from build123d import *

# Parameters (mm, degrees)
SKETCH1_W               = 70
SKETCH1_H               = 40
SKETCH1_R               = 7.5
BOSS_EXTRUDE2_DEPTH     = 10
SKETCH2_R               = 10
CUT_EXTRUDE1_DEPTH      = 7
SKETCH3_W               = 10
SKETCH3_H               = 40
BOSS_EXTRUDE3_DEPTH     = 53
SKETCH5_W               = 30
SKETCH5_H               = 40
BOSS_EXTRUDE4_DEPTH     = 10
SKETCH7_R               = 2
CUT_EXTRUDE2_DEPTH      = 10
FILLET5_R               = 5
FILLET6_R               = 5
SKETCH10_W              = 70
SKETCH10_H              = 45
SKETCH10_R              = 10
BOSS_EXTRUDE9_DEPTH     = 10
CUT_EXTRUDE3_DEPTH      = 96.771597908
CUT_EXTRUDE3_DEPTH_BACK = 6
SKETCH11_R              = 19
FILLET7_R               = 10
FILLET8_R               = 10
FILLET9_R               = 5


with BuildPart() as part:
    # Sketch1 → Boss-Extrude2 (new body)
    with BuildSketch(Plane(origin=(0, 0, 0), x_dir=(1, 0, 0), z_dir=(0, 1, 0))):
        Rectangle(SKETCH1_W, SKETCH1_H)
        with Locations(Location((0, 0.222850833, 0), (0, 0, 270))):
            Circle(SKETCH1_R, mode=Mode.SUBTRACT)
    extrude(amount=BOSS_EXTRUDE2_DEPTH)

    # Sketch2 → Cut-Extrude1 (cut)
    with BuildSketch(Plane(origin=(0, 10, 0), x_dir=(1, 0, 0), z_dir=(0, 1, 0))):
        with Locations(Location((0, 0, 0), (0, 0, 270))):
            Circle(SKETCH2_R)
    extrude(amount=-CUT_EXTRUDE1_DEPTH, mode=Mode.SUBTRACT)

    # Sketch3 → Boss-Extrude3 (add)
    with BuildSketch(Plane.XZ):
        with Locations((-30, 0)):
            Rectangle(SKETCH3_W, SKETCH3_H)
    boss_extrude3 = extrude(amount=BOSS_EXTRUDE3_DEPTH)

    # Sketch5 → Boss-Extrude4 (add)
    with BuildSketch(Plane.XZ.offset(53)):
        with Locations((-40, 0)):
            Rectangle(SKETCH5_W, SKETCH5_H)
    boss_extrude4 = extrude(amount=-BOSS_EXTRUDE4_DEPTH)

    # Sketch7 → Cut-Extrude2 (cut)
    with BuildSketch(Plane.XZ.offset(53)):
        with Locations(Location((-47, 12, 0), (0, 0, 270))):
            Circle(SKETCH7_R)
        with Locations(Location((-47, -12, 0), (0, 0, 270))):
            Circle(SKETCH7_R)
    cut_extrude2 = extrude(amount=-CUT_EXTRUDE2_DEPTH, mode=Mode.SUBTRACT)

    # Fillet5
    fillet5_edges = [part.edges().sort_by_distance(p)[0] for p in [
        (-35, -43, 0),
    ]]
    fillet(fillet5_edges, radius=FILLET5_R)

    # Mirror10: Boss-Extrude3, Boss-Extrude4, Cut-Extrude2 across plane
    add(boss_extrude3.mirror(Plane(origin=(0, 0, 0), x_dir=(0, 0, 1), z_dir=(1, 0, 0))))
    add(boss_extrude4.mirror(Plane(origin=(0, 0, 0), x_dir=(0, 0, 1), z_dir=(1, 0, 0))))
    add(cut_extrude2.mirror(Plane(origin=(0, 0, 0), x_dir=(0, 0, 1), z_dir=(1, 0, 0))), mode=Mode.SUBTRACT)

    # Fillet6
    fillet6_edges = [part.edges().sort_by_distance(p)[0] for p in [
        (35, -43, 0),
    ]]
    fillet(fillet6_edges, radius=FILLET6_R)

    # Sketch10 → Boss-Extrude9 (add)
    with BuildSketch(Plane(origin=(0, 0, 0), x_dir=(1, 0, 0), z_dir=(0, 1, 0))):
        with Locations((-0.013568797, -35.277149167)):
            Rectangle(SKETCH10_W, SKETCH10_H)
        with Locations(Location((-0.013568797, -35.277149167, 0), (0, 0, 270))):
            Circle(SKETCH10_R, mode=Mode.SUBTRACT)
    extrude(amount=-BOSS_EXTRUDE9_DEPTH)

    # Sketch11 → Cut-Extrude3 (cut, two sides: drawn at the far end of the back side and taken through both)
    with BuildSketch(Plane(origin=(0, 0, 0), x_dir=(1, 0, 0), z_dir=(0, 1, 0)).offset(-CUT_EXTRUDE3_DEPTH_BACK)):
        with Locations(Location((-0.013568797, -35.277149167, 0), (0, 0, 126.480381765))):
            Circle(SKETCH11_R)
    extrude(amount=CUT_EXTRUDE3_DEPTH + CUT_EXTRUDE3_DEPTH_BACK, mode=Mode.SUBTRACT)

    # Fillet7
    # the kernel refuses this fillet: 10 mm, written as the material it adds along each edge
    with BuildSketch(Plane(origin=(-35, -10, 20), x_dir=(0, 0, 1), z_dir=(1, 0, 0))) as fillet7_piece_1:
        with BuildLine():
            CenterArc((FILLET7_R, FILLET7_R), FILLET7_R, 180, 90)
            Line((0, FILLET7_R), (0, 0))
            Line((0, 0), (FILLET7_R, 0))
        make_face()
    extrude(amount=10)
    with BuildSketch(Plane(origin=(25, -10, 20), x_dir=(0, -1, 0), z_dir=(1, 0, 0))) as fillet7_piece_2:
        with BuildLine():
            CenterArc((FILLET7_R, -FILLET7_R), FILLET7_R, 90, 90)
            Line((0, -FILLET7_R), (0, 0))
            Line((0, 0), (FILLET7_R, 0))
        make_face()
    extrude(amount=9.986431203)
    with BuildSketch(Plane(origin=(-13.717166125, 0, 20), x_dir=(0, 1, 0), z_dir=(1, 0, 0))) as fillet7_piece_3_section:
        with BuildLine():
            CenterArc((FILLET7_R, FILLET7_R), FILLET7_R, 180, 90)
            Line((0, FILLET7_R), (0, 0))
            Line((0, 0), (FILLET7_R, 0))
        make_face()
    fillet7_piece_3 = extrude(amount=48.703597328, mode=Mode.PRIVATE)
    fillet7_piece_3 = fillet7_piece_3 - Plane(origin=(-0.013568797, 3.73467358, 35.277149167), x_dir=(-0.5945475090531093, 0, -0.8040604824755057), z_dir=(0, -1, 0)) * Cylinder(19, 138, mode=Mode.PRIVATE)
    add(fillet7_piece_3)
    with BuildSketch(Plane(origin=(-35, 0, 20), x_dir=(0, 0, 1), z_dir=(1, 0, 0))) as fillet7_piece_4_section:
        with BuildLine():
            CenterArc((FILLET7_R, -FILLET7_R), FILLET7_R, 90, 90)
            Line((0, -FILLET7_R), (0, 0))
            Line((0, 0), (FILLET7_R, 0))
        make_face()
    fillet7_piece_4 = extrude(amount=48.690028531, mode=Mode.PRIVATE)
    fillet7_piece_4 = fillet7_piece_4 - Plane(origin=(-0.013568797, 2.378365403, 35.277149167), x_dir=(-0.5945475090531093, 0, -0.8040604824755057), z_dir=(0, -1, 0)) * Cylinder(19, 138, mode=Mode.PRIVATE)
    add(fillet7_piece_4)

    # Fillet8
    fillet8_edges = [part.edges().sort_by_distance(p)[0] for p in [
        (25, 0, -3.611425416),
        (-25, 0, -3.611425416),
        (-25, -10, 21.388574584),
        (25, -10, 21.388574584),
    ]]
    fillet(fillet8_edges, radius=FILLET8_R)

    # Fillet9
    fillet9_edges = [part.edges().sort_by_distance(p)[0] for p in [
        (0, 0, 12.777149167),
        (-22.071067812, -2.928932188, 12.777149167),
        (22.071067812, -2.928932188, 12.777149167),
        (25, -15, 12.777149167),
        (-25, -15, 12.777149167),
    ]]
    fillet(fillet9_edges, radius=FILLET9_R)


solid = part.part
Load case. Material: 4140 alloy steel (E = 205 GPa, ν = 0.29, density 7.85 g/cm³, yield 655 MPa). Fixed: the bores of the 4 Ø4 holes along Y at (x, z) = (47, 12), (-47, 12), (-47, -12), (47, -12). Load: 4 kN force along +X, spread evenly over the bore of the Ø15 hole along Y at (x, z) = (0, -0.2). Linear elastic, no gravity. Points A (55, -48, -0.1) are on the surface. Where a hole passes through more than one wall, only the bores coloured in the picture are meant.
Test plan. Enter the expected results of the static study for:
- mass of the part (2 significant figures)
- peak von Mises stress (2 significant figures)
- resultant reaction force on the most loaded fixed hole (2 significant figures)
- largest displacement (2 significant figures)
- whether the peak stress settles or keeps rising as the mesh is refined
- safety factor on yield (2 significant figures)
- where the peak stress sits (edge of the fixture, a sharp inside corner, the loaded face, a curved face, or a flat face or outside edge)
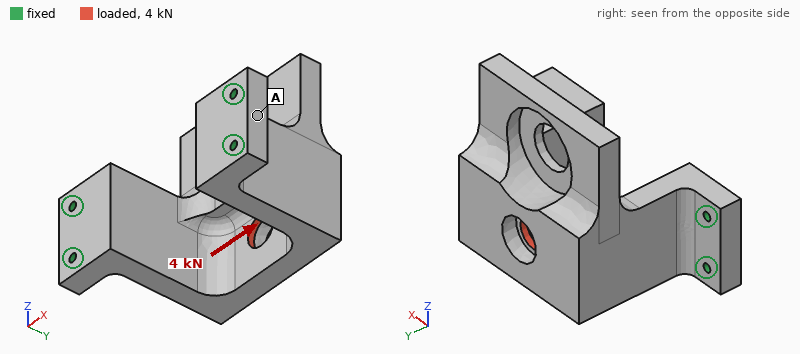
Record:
850 g
91 MPa
1.9 kN
37 µm
settles
7.2
a curved face
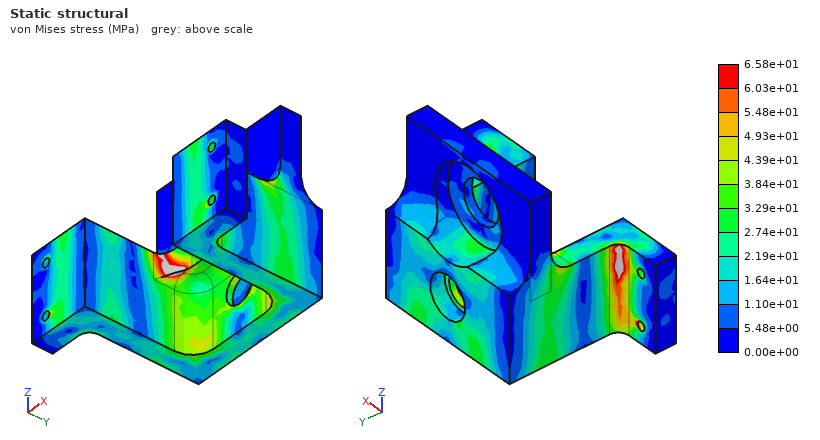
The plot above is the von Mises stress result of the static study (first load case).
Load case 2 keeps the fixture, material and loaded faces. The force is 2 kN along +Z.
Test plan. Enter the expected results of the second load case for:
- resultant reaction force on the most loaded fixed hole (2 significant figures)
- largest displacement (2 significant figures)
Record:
1.9 kN
31 µm
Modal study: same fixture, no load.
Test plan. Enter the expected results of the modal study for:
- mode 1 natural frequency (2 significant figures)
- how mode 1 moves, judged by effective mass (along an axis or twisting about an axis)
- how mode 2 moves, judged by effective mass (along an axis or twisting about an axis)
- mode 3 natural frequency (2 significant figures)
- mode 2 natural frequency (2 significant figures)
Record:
2000 Hz
along Z
along X
3000 Hz
2500 Hz
